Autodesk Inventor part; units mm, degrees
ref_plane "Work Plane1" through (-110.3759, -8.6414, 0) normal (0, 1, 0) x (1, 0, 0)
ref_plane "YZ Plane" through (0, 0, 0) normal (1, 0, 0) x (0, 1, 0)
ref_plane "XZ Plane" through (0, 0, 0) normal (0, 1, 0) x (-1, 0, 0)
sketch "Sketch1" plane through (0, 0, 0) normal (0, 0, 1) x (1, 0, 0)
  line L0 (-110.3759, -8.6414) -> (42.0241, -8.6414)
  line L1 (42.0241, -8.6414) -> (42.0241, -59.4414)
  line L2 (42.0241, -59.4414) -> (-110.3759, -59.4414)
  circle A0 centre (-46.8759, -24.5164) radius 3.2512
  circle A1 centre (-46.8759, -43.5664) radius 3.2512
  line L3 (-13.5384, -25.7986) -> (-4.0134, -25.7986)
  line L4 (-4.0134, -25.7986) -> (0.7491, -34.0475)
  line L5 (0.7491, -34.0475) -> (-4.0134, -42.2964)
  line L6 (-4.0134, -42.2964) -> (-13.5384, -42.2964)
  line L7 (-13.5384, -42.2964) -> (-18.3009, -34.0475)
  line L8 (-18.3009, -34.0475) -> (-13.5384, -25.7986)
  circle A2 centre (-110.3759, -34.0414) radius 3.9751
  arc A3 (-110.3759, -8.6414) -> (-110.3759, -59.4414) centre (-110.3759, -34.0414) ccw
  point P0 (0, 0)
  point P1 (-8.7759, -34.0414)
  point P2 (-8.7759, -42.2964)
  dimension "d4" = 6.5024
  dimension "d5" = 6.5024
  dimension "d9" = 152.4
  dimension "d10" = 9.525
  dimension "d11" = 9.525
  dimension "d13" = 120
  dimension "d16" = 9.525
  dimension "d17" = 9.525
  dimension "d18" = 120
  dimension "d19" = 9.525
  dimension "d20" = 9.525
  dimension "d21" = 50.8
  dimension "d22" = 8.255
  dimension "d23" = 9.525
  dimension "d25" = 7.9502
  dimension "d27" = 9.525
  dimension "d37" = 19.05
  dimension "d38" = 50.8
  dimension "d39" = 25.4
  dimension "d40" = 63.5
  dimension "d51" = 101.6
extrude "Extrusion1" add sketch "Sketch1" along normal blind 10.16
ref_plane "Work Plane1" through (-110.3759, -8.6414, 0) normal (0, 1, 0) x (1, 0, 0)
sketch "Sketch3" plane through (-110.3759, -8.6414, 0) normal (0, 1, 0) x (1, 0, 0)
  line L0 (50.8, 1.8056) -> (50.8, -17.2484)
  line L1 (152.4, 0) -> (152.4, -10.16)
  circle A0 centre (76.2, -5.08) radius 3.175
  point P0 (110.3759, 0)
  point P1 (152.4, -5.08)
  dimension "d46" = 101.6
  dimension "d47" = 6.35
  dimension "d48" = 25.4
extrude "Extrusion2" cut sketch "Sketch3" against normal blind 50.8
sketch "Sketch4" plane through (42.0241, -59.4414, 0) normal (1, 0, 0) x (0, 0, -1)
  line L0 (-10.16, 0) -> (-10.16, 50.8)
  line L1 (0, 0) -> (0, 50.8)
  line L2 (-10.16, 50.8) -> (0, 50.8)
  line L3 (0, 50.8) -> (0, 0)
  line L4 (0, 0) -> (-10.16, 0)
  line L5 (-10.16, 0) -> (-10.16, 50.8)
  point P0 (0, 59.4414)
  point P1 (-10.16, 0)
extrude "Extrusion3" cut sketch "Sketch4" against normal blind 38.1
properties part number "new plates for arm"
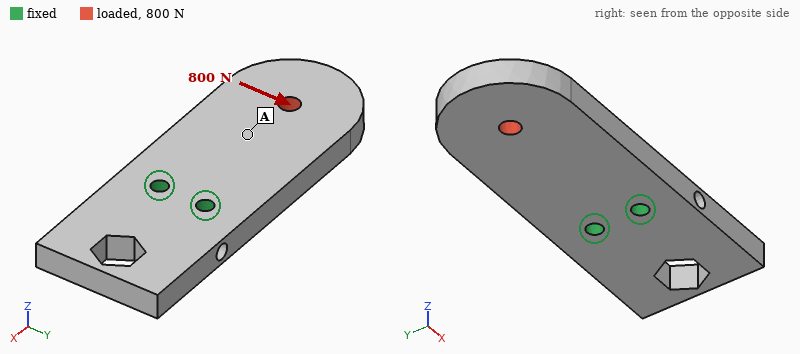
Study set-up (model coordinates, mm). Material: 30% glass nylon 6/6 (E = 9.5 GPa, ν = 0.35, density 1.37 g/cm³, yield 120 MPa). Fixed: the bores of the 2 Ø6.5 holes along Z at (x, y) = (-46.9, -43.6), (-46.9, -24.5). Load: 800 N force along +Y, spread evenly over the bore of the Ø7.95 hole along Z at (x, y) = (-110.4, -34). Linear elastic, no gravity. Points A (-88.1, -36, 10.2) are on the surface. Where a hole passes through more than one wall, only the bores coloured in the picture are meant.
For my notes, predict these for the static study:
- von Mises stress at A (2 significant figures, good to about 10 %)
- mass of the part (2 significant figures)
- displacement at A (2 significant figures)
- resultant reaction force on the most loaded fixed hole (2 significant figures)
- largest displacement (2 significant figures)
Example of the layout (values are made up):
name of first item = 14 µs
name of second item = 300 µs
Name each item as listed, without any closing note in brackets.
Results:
von Mises stress at A = 4.1 MPa
mass of the part = 88 g
displacement at A = 0.086 mm
resultant reaction force on the most loaded fixed hole = 2.1 kN
largest displacement = 0.21 mm
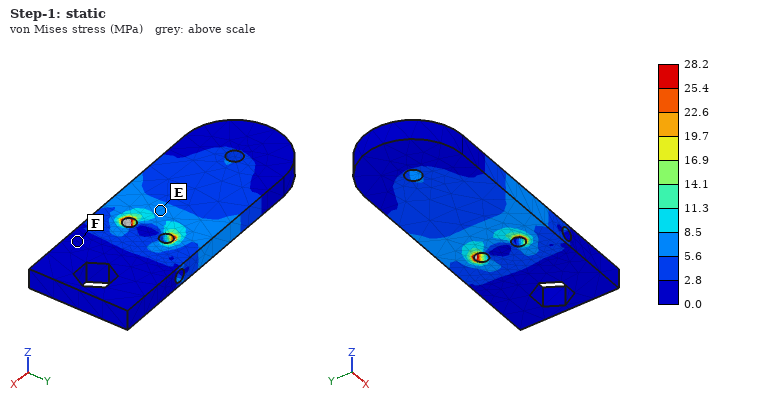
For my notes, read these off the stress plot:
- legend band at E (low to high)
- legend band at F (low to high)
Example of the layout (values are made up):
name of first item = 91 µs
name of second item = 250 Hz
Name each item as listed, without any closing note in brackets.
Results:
legend band at E = 5.6 to 8.5 MPa
legend band at F = 0.0 to 2.8 MPa
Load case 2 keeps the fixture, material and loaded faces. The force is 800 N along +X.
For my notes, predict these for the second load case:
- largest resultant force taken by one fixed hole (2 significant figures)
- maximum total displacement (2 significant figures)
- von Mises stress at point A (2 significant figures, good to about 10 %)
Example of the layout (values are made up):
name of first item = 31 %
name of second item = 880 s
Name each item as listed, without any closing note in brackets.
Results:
largest resultant force taken by one fixed hole = 400 N
maximum total displacement = 15 µm
von Mises stress at point A = 2.1 MPa
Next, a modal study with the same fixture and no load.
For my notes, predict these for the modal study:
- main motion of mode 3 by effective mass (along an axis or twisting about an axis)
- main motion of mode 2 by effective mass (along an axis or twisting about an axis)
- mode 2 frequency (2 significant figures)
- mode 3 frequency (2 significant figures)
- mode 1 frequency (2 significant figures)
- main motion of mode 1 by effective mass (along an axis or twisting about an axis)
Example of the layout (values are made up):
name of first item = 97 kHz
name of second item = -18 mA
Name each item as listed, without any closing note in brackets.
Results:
main motion of mode 3 by effective mass = along Y
main motion of mode 2 by effective mass = along Z
mode 2 frequency = 1700 Hz
mode 3 frequency = 1900 Hz
mode 1 frequency = 620 Hz
main motion of mode 1 by effective mass = along Z
